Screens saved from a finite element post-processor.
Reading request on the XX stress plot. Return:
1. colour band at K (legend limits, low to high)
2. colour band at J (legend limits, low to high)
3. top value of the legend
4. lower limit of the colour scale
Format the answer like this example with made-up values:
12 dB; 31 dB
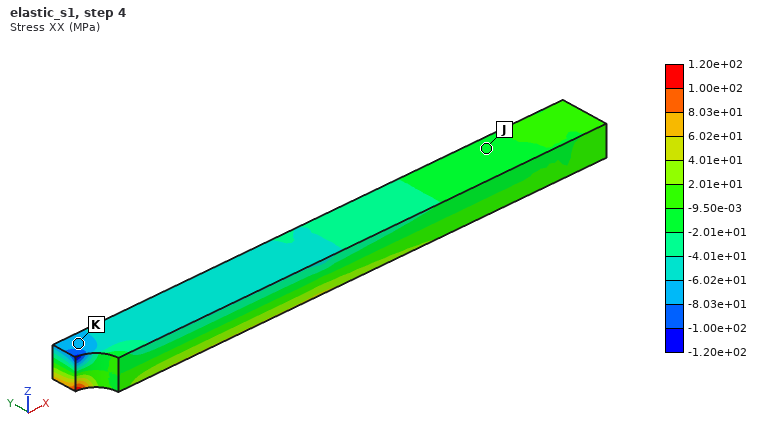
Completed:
-8.03e+01 to -6.02e+01 MPa; -2.01e+01 to -9.50e-03 MPa; 1.20e+02 MPa; -1.20e+02 MPa
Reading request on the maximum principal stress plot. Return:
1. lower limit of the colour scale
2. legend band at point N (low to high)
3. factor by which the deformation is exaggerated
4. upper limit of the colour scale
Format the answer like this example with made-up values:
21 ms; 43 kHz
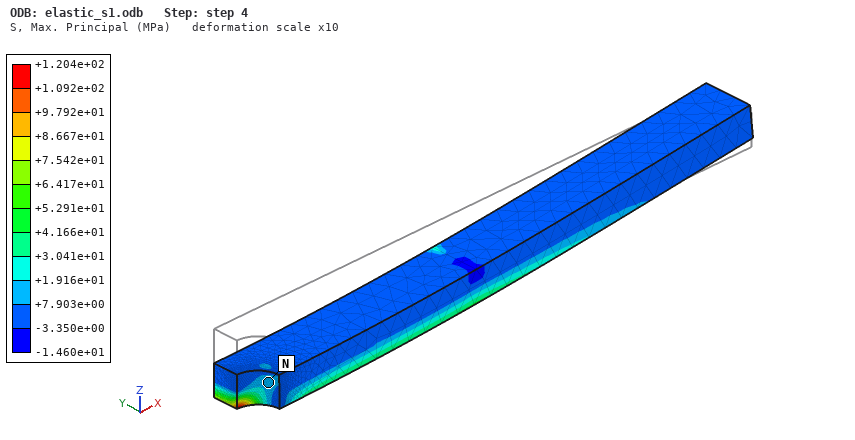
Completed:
-1.460e+01 MPa; +7.903e+00 to +1.916e+01 MPa; 10; +1.204e+02 MPa
